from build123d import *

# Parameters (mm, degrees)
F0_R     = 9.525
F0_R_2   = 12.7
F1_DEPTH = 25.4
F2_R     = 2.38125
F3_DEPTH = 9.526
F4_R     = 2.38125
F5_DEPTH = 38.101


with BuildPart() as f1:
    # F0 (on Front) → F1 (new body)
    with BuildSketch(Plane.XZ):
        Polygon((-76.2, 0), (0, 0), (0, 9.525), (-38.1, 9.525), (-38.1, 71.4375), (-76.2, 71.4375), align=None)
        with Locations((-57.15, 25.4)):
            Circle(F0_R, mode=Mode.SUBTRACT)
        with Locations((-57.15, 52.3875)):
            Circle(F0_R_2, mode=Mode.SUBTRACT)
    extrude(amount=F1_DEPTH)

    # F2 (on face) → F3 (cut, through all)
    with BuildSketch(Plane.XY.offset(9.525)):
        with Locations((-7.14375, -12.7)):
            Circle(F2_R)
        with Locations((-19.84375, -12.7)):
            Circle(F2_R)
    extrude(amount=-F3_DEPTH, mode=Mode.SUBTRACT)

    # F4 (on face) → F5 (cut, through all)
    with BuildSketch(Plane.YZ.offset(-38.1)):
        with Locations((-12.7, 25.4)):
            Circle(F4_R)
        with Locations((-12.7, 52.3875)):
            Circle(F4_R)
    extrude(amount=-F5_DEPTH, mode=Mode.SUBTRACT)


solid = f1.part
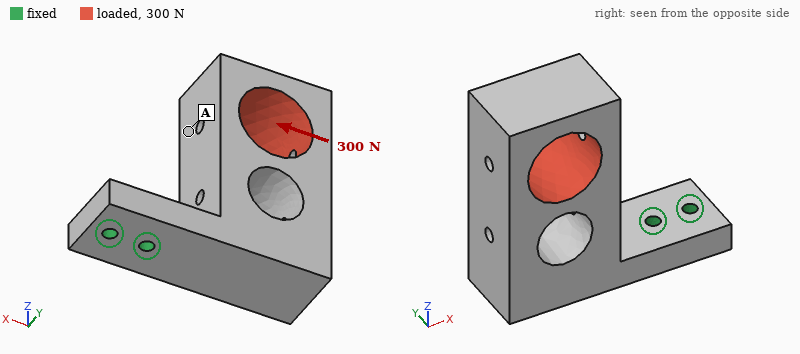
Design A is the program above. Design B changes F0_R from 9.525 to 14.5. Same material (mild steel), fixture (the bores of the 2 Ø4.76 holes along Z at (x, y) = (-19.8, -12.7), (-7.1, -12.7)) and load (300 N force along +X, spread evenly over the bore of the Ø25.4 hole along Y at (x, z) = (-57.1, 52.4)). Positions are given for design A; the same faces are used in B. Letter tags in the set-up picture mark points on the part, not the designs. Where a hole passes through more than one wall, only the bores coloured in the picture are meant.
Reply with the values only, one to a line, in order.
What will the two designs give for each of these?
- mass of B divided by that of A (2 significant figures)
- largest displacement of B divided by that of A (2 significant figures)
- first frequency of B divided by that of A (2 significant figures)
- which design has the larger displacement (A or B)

0.84
1.2
1.0
B
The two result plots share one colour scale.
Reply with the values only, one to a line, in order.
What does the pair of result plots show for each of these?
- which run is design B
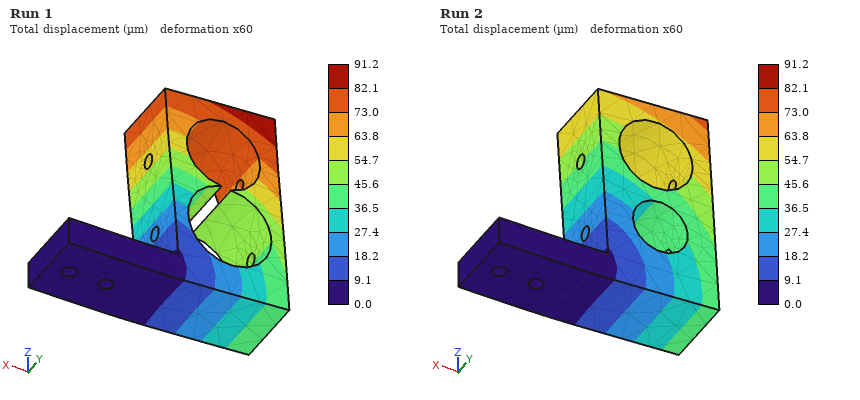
Run 1
